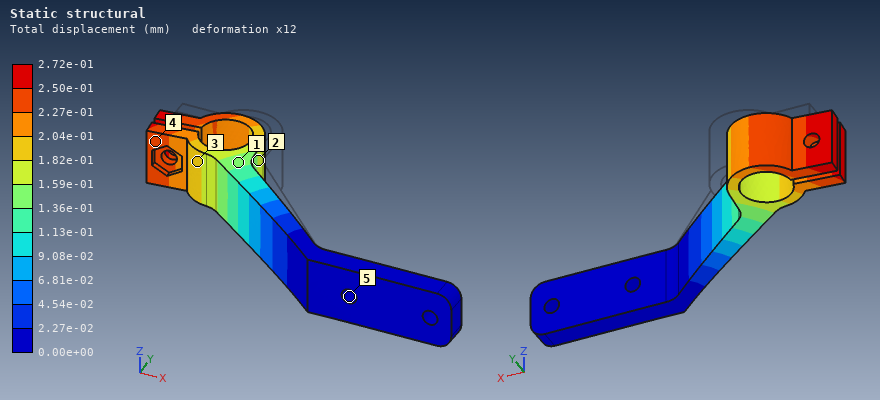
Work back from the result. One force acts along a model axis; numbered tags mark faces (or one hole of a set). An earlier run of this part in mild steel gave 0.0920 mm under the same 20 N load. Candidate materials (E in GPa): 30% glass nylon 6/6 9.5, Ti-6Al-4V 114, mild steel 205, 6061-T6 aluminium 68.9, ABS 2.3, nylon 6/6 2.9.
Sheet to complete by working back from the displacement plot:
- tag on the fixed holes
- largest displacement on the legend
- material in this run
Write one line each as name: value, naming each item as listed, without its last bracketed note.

tag on the fixed holes: 5
largest displacement on the legend: 2.72e-01 mm
material in this run: 6061-T6 aluminium
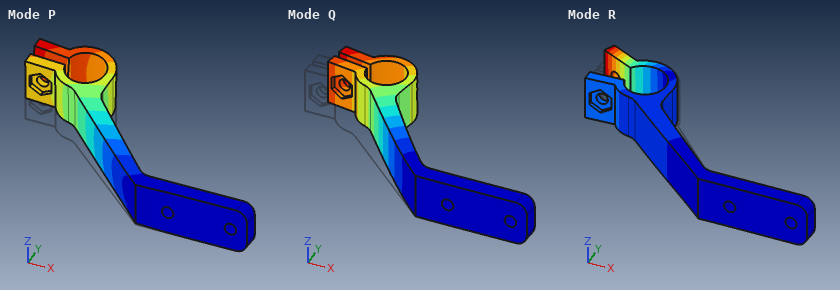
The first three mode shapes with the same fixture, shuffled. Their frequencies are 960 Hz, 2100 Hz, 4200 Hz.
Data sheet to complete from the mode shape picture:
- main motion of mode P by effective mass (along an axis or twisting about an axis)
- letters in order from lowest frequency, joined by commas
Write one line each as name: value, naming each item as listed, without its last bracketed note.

main motion of mode P by effective mass: along Z
letters in order from lowest frequency, joined by commas: Q, P, R
